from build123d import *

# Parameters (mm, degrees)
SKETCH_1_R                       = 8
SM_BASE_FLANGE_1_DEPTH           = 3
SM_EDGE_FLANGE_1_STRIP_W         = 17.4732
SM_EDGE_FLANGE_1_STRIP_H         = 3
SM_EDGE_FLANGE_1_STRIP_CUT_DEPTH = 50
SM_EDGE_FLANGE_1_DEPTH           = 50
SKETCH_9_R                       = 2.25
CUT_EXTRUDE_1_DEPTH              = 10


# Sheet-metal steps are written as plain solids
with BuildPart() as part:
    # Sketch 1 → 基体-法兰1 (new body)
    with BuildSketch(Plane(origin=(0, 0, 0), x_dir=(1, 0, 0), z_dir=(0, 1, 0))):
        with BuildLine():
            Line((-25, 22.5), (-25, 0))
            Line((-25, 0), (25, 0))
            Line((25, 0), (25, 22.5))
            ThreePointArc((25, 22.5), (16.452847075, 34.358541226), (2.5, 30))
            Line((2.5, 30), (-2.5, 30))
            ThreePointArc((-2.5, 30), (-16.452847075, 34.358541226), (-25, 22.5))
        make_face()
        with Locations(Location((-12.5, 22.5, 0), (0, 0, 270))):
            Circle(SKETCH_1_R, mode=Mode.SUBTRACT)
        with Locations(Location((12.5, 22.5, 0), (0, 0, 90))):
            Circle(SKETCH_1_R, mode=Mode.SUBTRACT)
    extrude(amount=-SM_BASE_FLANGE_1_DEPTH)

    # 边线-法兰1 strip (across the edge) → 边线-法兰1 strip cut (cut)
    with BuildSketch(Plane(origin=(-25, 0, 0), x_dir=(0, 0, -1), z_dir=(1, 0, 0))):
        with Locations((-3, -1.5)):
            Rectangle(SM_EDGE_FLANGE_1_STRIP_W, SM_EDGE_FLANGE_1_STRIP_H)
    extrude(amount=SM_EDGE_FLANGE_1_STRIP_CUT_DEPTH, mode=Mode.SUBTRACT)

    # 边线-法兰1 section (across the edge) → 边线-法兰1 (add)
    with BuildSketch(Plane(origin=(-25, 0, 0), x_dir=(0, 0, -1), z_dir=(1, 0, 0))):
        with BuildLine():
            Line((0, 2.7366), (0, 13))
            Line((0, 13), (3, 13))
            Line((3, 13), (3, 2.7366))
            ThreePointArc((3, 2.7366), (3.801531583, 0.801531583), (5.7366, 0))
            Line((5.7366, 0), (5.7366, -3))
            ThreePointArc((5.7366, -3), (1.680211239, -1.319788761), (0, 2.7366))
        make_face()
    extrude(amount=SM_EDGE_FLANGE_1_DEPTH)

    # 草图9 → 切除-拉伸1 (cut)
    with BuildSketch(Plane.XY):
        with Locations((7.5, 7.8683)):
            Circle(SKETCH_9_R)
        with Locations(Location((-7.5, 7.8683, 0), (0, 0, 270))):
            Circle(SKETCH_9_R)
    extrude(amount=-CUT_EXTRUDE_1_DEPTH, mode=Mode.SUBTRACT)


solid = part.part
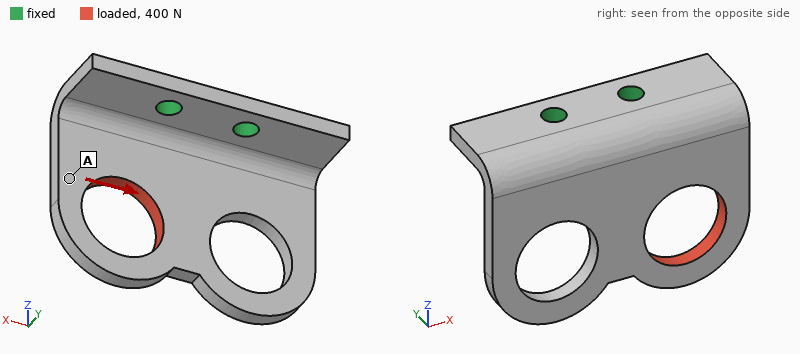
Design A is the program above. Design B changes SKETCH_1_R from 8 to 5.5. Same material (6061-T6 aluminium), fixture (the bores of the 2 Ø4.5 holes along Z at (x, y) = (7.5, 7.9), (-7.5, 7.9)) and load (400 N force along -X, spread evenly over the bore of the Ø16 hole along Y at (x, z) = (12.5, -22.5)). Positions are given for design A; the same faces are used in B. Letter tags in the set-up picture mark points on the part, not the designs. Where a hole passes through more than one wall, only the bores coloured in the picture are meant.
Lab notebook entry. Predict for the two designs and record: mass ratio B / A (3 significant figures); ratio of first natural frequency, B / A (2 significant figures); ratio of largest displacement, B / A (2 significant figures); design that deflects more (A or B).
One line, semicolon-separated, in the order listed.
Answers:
1.12; 0.91; 0.90; A
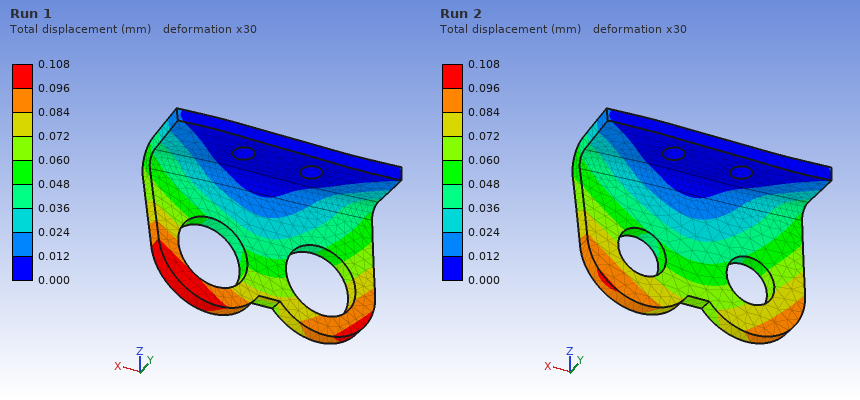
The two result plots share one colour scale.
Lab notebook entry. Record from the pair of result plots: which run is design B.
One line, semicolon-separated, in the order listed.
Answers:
Run 2
